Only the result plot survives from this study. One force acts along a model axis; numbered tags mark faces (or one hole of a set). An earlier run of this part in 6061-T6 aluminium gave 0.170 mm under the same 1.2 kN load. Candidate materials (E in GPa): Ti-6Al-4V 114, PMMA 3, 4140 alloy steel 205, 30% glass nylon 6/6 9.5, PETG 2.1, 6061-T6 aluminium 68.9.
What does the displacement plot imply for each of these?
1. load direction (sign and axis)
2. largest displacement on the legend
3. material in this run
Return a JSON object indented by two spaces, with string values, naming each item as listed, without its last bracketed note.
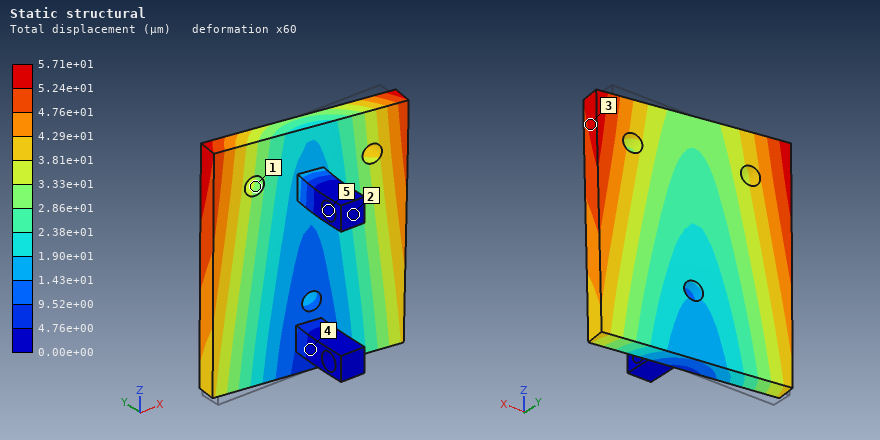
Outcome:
{
  "load direction": "+X",
  "largest displacement on the legend": "5.71e+01 µm",
  "material in this run": "4140 alloy steel"
}
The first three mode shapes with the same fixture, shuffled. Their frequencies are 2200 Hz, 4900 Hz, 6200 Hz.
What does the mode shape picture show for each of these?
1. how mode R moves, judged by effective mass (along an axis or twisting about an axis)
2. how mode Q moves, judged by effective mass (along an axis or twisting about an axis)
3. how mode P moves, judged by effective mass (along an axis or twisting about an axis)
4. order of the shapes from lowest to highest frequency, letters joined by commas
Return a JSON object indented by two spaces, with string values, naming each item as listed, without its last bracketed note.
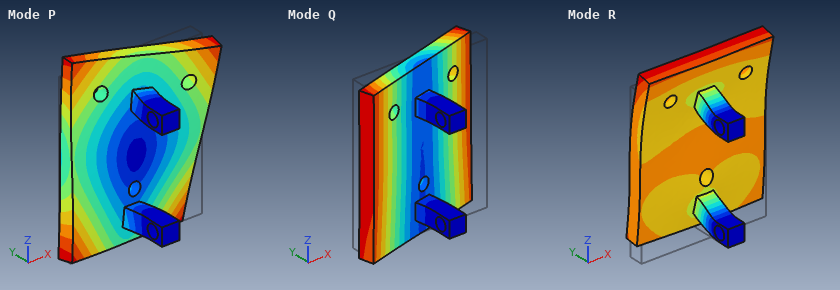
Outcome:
{
  "how mode R moves, judged by effective mass": "along Z",
  "how mode Q moves, judged by effective mass": "along X",
  "how mode P moves, judged by effective mass": "twisting about Y",
  "order of the shapes from lowest to highest frequency, letters joined by commas": "Q, P, R"
}
